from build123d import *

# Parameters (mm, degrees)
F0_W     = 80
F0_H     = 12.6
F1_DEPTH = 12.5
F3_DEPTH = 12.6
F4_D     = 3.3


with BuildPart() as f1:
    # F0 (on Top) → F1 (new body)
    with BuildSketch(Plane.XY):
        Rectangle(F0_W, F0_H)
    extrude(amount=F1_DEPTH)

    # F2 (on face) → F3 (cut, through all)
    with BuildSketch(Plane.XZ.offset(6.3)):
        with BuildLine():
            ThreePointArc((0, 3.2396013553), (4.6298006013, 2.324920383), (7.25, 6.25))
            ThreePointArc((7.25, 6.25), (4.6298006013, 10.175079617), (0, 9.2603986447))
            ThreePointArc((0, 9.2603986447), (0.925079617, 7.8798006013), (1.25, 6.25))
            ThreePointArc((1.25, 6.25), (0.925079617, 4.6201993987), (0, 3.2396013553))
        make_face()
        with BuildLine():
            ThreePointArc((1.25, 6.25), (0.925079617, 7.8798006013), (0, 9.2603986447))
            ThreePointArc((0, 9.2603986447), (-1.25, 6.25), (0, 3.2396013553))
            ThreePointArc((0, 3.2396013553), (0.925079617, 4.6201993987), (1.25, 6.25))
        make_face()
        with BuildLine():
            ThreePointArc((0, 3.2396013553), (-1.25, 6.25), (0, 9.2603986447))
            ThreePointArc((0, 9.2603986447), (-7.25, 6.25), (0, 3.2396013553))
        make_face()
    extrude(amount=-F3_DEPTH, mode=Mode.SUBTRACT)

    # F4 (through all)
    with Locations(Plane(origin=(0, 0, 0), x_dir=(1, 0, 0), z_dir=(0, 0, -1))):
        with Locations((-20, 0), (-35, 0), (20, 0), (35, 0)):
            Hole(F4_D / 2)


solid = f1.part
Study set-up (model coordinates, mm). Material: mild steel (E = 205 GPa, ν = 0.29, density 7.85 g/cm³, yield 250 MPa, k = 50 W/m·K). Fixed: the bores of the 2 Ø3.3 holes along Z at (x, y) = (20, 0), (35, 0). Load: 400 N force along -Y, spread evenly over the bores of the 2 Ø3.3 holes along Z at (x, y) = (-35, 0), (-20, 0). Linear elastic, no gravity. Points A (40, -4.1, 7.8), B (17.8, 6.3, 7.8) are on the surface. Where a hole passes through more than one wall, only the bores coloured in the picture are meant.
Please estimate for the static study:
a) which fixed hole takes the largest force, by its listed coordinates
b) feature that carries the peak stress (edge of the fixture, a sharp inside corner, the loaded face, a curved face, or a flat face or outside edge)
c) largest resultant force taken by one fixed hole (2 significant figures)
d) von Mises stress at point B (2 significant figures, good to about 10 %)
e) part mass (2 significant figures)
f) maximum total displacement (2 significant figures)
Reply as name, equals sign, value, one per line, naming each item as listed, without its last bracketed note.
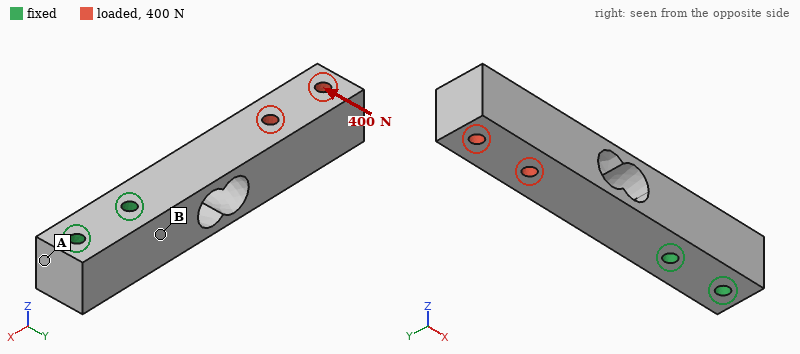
which fixed hole takes the largest force, by its listed coordinates = (20, 0)
feature that carries the peak stress = a curved face
largest resultant force taken by one fixed hole = 1.2 kN
von Mises stress at point B = 49 MPa
part mass = 85 g
maximum total displacement = 96 µm
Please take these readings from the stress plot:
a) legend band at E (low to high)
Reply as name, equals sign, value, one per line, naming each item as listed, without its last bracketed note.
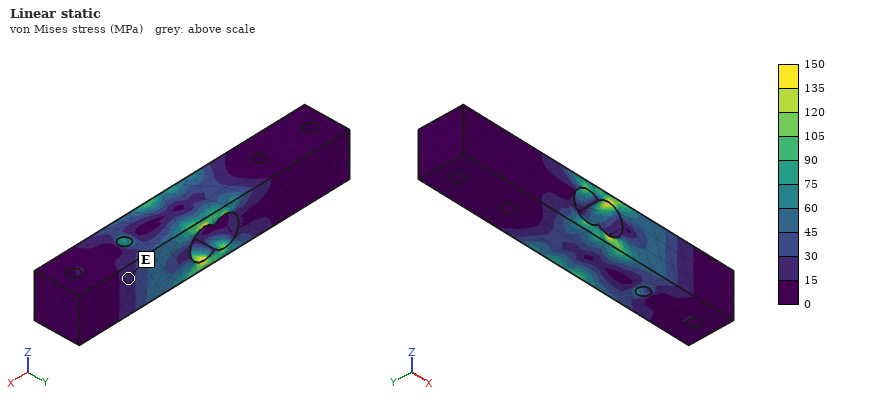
legend band at E = 15 to 30 MPa
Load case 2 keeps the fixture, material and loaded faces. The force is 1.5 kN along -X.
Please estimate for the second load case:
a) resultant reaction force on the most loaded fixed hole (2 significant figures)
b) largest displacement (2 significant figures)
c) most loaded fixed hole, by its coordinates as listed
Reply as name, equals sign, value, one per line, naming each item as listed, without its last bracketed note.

resultant reaction force on the most loaded fixed hole = 1.3 kN
largest displacement = 4.2 µm
most loaded fixed hole, by its coordinates as listed = (20, 0)
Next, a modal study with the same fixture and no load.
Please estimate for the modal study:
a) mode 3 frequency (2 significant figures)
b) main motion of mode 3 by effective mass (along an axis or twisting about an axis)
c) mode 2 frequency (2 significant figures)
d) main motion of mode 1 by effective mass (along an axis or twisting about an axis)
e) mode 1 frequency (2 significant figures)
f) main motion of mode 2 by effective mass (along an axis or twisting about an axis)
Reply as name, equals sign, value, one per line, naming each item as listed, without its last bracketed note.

mode 3 frequency = 8400 Hz
main motion of mode 3 by effective mass = twisting about X
mode 2 frequency = 2200 Hz
main motion of mode 1 by effective mass = along Y
mode 1 frequency = 2100 Hz
main motion of mode 2 by effective mass = along Z
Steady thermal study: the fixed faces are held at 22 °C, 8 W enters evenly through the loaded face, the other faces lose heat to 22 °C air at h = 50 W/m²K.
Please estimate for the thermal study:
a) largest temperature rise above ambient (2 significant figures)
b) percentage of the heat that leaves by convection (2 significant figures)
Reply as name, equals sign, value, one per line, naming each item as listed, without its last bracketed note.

largest temperature rise above ambient = 42 K
percentage of the heat that leaves by convection = 52 %
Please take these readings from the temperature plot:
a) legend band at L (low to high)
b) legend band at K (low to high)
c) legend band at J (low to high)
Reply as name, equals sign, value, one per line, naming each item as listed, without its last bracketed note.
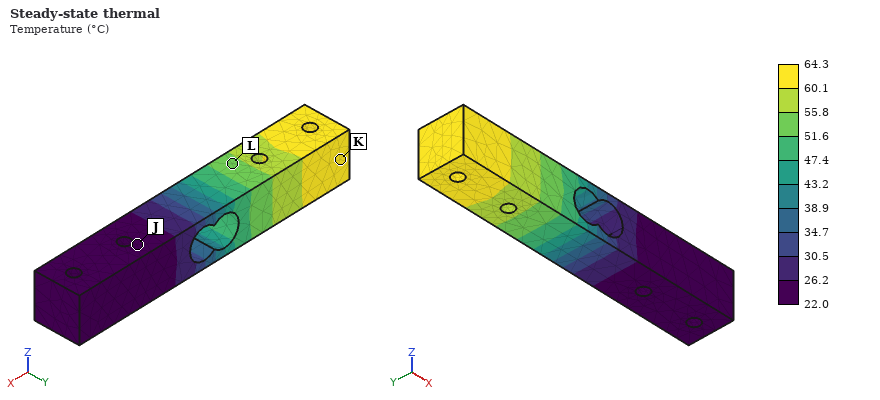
legend band at L = 51.6 to 55.8 °C
legend band at K = 60.1 to 64.3 °C
legend band at J = 22.0 to 26.2 °C
